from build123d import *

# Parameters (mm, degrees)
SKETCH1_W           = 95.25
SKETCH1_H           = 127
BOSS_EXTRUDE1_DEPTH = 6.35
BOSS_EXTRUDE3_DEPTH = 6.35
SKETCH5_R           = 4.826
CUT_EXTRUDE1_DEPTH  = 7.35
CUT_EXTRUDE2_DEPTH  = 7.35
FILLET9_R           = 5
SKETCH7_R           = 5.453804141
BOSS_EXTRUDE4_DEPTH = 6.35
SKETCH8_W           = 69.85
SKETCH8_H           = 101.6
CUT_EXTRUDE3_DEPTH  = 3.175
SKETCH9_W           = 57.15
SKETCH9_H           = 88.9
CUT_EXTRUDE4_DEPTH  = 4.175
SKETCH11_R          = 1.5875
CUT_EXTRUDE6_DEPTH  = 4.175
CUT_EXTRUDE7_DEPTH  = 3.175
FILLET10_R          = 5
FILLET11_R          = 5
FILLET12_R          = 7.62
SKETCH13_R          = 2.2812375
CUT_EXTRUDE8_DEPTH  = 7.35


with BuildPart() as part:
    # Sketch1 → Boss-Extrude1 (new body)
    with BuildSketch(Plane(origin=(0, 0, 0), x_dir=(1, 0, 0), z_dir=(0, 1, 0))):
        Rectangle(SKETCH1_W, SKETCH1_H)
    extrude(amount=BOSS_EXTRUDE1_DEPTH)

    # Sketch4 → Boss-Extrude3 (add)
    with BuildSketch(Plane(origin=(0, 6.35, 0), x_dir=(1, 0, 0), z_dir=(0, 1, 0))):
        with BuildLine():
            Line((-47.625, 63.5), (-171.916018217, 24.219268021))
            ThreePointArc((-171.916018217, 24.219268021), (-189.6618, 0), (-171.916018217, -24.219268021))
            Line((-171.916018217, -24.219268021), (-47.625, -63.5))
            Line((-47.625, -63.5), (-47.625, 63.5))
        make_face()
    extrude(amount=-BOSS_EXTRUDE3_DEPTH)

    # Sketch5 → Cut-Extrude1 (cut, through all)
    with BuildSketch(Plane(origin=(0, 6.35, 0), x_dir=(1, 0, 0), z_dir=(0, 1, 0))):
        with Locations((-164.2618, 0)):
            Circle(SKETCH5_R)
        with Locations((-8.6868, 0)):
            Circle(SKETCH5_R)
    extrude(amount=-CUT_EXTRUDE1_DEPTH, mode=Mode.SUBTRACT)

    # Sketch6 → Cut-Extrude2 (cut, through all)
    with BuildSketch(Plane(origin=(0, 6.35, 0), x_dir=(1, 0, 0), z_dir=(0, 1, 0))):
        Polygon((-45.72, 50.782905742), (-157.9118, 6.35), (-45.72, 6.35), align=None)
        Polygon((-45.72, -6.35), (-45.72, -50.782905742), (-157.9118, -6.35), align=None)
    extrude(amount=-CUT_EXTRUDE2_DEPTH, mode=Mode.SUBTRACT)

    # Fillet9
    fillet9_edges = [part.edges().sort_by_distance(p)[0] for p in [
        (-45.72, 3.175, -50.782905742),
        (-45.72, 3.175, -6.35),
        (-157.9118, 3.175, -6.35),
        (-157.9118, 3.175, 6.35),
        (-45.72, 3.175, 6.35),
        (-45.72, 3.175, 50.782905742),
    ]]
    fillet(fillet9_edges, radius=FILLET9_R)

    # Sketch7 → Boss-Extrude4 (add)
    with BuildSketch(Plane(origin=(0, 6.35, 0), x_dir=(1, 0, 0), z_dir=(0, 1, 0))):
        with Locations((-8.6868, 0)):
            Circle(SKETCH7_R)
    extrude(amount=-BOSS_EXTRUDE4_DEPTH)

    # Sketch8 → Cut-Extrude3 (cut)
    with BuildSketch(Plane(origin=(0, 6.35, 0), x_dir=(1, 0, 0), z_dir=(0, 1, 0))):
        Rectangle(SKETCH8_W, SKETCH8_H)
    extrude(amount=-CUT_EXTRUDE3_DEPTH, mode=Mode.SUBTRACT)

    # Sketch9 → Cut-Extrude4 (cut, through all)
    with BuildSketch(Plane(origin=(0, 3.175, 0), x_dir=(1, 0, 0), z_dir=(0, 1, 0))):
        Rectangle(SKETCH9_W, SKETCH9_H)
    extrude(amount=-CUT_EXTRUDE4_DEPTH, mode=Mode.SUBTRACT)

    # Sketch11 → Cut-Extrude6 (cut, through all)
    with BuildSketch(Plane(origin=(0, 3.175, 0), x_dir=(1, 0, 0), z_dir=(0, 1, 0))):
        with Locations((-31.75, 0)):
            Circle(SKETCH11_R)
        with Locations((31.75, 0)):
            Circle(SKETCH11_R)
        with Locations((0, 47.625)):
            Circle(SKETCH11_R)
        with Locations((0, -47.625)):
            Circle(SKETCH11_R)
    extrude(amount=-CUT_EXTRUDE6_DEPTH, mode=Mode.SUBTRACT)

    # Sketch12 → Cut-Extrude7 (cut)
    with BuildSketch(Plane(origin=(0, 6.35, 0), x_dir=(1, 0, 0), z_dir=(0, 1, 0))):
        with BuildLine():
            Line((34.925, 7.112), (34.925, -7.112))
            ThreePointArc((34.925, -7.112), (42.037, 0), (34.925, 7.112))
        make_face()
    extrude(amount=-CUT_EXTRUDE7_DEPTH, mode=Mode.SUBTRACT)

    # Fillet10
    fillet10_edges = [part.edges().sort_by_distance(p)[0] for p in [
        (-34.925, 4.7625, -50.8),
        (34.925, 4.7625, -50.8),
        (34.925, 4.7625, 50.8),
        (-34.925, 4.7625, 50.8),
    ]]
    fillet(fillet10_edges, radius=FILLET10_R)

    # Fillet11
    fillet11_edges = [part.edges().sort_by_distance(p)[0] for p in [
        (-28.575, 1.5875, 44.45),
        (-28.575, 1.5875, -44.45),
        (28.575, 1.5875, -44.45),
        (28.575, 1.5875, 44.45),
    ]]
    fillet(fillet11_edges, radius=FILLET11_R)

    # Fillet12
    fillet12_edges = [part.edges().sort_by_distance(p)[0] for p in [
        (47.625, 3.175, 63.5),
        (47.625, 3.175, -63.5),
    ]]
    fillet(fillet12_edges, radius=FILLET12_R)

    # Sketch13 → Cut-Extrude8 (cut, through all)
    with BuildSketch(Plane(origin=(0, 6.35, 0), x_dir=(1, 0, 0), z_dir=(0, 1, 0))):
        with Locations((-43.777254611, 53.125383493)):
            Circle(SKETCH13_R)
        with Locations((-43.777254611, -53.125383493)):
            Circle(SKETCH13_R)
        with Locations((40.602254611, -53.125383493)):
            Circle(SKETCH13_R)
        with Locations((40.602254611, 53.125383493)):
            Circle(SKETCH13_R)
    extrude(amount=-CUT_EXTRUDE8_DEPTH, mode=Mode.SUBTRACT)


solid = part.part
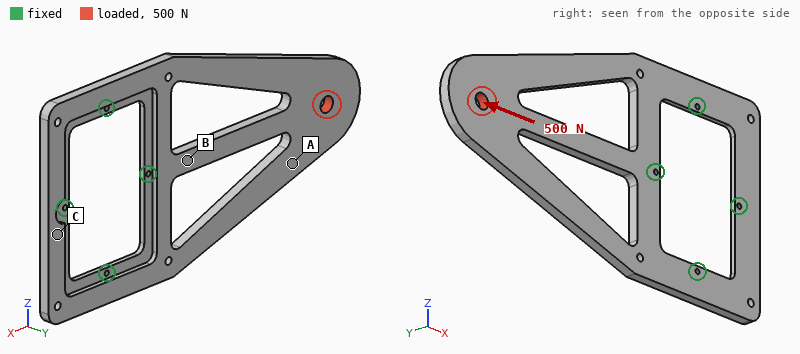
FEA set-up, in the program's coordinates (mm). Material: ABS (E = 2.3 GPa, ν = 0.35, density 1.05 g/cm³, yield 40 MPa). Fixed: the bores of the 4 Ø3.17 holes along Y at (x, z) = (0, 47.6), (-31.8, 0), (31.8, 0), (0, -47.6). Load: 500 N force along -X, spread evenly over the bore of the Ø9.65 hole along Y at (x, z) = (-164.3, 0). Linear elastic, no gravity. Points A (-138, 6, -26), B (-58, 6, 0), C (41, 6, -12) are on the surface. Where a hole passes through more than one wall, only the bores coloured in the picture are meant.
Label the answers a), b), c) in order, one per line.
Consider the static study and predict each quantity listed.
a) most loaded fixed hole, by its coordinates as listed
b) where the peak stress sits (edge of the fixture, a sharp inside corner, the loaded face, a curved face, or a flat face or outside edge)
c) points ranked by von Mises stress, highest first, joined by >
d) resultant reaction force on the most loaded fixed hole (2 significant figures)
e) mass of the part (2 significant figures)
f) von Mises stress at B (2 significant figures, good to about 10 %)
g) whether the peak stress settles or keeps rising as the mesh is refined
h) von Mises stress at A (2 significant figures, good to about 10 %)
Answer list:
a) (-31.8, 0)
b) edge of the fixture
c) B > A > C
d) 190 N
e) 84 g
f) 2.2 MPa
g) keeps rising
h) 1.3 MPa
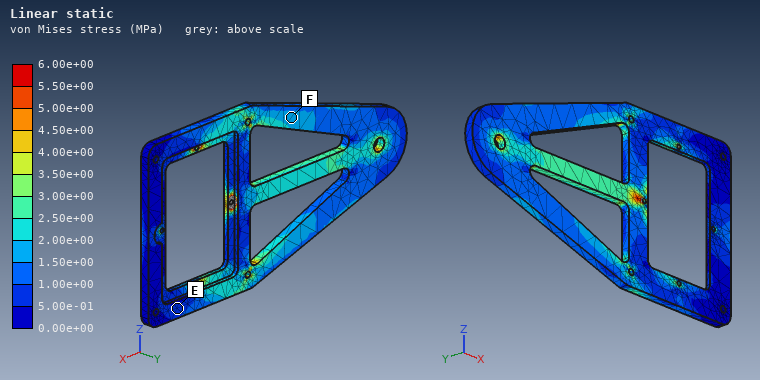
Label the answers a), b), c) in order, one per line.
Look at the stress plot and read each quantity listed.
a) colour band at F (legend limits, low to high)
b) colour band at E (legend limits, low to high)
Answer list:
a) 1.50e+00 to 2.00e+00 MPa
b) 5.00e-01 to 1.00e+00 MPa
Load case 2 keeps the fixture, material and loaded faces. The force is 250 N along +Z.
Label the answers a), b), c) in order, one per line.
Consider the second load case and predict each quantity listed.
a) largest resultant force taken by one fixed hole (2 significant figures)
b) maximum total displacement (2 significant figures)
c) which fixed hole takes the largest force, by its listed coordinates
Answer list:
a) 330 N
b) 0.86 mm
c) (-31.8, 0)
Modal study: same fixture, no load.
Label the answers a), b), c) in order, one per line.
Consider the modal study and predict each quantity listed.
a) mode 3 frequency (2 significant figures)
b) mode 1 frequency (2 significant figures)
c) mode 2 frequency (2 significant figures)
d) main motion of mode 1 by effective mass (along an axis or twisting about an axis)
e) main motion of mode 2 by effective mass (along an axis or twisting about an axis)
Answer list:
a) 280 Hz
b) 44 Hz
c) 180 Hz
d) along Y
e) twisting about X
